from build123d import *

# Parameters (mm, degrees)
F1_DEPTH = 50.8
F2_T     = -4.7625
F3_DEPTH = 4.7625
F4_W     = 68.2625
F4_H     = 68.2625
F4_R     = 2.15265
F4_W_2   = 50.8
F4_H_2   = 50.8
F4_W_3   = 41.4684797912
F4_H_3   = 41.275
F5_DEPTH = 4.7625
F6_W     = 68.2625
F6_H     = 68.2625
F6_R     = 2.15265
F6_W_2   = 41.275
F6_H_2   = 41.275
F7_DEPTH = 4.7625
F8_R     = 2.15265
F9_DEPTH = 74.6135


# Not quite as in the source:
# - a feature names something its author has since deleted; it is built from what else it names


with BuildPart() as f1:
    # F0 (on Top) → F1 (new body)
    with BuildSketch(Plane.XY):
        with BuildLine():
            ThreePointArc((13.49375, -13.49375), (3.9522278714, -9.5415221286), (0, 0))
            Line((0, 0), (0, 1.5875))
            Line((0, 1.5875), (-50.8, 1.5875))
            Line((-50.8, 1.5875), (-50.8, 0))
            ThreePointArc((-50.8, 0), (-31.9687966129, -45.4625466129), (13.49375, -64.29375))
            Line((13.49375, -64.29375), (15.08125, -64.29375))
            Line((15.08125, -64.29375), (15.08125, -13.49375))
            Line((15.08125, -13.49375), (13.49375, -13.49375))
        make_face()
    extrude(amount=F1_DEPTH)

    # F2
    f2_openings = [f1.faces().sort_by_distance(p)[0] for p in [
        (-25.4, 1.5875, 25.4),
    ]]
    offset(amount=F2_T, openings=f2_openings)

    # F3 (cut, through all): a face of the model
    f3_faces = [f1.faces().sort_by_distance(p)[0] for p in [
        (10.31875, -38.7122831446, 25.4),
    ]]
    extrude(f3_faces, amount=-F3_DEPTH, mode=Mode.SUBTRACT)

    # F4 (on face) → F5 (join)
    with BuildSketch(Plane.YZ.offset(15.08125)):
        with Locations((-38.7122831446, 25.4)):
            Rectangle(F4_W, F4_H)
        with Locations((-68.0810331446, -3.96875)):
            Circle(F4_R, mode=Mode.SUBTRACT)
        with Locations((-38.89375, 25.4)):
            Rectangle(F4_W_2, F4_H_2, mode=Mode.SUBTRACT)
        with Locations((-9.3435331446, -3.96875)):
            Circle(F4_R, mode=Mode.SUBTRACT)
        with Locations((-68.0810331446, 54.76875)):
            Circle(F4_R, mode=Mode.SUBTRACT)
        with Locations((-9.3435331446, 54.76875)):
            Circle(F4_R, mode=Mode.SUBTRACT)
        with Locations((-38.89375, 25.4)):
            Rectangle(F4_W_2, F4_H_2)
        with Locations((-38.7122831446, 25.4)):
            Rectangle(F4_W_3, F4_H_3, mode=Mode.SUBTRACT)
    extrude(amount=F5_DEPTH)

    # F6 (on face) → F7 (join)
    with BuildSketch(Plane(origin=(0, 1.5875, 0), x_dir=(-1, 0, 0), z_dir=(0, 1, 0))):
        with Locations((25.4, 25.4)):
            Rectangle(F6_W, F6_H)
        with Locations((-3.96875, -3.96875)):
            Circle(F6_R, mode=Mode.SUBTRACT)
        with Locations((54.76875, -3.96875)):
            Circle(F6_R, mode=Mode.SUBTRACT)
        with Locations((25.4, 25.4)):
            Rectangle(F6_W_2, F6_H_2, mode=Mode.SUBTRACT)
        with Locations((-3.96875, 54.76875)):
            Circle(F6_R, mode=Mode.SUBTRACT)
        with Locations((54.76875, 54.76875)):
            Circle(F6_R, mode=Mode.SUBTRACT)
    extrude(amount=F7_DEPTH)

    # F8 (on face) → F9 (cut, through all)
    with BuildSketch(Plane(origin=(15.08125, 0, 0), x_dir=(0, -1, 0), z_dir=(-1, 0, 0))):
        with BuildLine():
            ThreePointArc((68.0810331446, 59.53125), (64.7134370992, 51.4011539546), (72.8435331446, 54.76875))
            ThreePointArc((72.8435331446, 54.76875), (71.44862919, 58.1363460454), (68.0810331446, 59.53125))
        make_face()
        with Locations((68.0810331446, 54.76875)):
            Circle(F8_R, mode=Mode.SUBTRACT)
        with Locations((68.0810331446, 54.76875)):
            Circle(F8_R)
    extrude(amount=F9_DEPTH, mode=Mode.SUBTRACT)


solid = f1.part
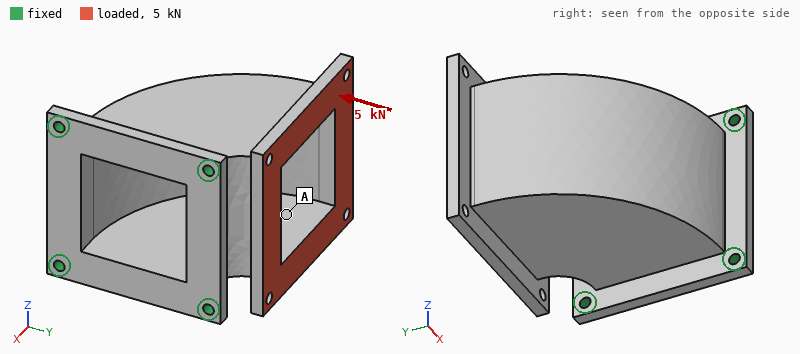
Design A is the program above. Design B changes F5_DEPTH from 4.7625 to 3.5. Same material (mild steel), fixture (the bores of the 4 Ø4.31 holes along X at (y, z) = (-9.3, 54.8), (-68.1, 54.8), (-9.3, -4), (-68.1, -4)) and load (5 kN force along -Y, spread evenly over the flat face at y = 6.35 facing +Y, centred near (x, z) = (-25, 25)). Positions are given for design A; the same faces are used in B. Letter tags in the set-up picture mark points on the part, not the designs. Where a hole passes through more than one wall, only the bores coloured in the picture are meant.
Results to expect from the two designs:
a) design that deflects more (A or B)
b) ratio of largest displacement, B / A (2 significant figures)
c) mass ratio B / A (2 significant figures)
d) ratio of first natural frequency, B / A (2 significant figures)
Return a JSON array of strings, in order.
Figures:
["B", "1.3", "0.96", "0.89"]
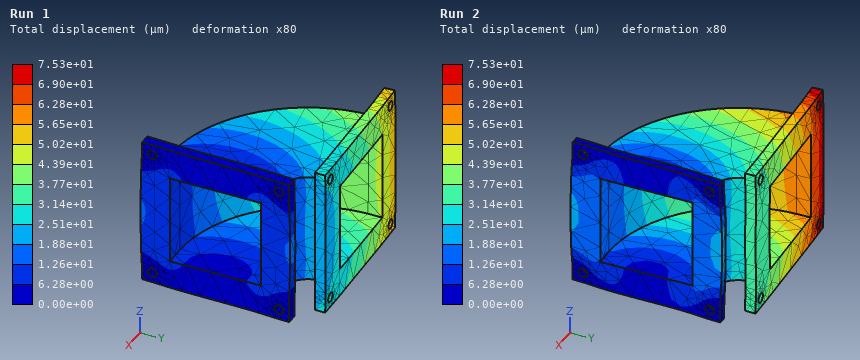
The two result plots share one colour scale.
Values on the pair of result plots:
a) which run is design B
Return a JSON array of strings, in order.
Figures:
["Run 2"]
